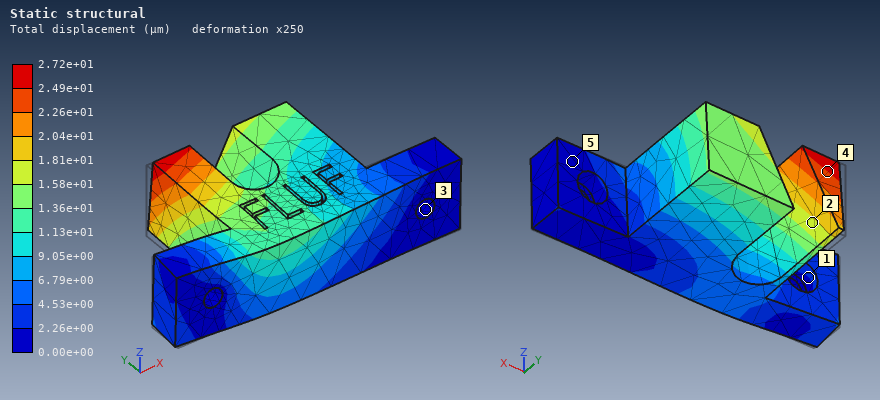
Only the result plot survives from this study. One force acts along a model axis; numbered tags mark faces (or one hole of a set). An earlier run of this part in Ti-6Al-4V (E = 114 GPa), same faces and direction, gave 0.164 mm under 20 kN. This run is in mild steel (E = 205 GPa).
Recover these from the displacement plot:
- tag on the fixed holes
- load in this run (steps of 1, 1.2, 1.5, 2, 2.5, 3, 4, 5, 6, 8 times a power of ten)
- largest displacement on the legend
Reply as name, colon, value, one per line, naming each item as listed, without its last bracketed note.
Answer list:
tag on the fixed holes: 3
load in this run: 6 kN
largest displacement on the legend: 2.72e+01 µm
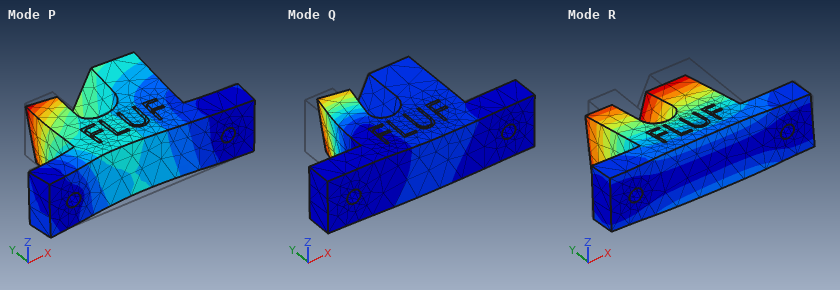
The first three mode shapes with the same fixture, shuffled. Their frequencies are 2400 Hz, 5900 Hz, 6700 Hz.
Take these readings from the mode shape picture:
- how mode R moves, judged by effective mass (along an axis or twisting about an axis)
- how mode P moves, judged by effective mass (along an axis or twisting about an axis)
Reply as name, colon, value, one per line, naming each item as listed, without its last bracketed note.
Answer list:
how mode R moves, judged by effective mass: along Z
how mode P moves, judged by effective mass: along Y
